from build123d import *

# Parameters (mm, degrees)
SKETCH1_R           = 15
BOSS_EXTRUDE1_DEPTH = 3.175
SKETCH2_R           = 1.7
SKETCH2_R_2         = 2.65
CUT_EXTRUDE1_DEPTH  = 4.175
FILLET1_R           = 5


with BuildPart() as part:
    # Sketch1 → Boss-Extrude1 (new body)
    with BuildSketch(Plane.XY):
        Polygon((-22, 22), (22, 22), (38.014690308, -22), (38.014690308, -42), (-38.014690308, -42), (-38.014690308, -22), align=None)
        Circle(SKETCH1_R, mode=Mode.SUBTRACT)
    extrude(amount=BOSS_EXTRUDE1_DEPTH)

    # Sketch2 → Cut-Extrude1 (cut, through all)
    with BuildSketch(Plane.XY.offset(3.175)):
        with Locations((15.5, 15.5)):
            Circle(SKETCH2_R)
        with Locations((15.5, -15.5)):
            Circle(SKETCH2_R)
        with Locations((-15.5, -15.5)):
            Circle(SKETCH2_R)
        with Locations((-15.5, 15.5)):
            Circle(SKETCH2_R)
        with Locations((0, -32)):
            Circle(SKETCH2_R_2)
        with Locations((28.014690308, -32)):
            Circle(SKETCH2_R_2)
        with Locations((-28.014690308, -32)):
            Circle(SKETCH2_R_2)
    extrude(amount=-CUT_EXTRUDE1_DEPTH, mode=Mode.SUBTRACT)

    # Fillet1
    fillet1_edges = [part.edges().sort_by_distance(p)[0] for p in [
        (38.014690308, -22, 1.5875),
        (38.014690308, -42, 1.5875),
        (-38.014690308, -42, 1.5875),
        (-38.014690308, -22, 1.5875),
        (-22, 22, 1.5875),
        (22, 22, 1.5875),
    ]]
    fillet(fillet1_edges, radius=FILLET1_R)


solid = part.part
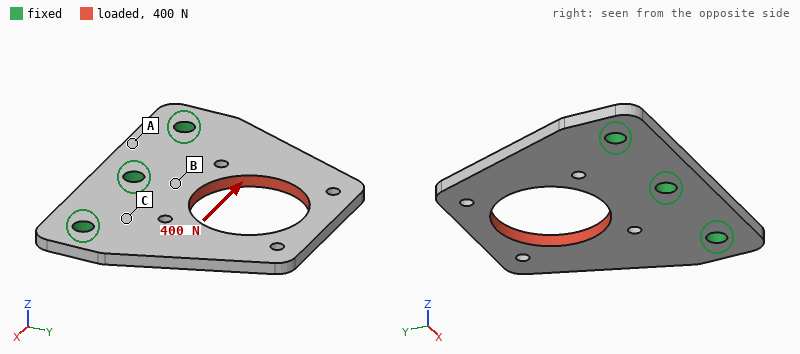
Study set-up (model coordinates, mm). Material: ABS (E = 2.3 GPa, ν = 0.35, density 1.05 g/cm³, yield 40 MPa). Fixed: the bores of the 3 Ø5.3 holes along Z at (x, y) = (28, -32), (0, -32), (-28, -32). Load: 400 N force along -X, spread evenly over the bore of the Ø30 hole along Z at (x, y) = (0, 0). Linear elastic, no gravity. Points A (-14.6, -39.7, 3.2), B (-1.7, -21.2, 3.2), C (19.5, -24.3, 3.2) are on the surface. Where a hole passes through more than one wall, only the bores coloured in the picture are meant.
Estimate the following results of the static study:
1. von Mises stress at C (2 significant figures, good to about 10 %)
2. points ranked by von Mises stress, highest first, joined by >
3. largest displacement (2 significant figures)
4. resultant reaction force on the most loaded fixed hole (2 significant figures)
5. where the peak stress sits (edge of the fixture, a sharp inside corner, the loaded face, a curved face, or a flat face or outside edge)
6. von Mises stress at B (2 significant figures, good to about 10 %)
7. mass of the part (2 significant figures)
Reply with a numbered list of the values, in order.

1. 2.6 MPa
2. B > C > A
3. 0.29 mm
4. 230 N
5. edge of the fixture
6. 5.8 MPa
7. 11 g
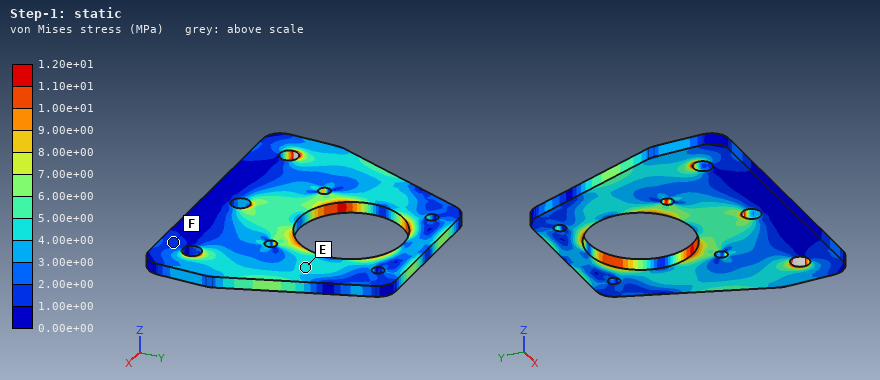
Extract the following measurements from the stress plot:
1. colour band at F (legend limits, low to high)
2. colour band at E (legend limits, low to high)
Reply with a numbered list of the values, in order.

1. 1.00e+00 to 2.00e+00 MPa
2. 4.00e+00 to 5.00e+00 MPa
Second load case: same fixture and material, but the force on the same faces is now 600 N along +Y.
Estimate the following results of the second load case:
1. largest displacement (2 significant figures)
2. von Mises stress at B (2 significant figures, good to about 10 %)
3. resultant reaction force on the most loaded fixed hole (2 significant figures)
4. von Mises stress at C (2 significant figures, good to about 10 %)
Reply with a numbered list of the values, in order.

1. 0.17 mm
2. 2.6 MPa
3. 230 N
4. 2.8 MPa
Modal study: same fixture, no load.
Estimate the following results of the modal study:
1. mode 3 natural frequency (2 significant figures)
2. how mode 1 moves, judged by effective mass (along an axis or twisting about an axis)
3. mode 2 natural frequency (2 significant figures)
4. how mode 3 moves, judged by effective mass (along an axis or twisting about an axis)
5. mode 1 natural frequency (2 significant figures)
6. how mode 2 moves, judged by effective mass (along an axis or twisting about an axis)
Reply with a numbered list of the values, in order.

1. 1500 Hz
2. along Z
3. 690 Hz
4. along Z
5. 330 Hz
6. twisting about Y
